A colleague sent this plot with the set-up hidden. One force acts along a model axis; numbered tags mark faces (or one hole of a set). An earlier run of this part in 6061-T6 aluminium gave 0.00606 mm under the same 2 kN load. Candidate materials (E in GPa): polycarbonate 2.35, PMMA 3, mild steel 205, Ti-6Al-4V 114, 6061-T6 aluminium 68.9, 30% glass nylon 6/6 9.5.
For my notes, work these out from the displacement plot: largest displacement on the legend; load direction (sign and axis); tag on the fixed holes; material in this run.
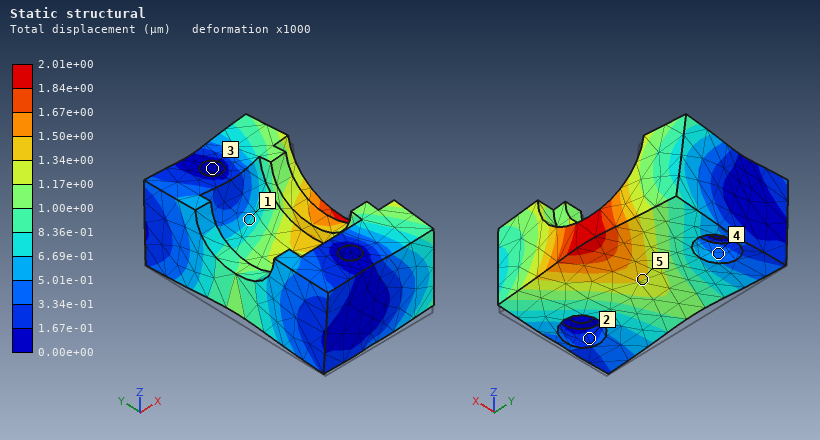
2.01e+00 µm
+Z
3
mild steel
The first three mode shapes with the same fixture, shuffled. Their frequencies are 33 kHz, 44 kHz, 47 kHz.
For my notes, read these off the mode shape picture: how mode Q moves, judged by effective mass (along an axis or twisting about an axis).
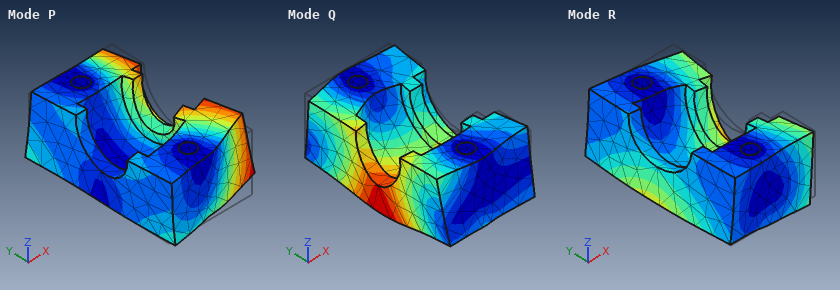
along Z
